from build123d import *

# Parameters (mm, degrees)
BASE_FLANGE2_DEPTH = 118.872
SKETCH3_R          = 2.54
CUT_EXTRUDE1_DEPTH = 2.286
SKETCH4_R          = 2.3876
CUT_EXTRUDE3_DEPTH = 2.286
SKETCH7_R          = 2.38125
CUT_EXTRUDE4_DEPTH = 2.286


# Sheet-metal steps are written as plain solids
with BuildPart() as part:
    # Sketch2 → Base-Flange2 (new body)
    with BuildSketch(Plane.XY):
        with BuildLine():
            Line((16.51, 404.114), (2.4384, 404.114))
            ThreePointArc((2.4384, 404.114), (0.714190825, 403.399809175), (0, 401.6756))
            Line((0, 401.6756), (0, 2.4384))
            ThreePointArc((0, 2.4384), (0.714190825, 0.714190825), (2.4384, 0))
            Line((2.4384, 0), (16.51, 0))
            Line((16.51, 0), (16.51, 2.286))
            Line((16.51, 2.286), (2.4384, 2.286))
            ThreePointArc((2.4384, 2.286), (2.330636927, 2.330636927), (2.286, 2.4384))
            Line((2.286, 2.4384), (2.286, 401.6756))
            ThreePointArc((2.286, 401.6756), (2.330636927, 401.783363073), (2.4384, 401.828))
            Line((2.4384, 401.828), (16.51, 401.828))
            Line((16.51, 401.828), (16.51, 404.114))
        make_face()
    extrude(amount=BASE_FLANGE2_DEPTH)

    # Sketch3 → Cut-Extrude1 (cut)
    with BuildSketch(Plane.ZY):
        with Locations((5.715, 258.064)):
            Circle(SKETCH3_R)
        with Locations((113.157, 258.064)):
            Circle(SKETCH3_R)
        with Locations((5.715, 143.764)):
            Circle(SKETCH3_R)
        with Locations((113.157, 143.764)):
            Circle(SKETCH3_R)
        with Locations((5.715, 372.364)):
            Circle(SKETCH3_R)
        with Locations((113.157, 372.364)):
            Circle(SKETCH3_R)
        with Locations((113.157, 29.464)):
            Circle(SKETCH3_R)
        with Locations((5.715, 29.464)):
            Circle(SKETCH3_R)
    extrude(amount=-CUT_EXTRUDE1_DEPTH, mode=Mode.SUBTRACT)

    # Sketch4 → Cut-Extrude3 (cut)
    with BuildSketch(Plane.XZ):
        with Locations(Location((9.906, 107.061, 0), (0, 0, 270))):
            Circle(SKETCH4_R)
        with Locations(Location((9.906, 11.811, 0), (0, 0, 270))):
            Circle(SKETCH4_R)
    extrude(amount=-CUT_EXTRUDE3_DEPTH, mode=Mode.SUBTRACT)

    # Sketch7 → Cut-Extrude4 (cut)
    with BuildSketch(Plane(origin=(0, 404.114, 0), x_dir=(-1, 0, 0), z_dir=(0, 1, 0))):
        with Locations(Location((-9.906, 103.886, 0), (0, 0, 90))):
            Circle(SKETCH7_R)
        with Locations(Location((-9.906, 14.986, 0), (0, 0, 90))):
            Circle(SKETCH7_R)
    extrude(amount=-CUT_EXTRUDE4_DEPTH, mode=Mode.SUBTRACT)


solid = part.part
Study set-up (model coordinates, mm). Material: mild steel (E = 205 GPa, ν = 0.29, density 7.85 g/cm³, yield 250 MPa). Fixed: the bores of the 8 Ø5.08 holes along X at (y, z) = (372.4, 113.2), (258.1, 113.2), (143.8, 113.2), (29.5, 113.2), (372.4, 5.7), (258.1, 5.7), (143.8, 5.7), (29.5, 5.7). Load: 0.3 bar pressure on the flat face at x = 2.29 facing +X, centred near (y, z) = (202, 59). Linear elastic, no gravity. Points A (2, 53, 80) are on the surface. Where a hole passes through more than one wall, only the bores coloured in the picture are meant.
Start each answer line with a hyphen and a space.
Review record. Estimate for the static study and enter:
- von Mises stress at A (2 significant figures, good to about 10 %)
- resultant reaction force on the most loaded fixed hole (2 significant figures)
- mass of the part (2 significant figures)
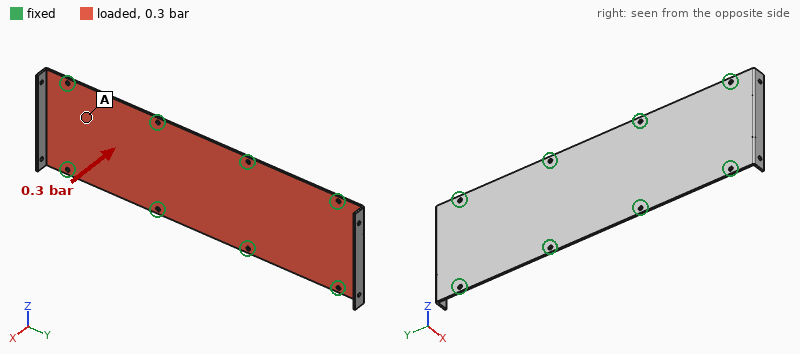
- 13 MPa
- 210 N
- 920 g
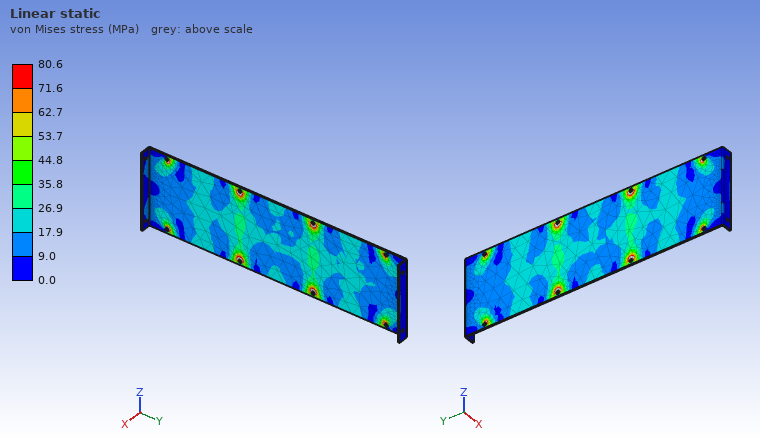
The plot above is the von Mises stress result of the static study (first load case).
